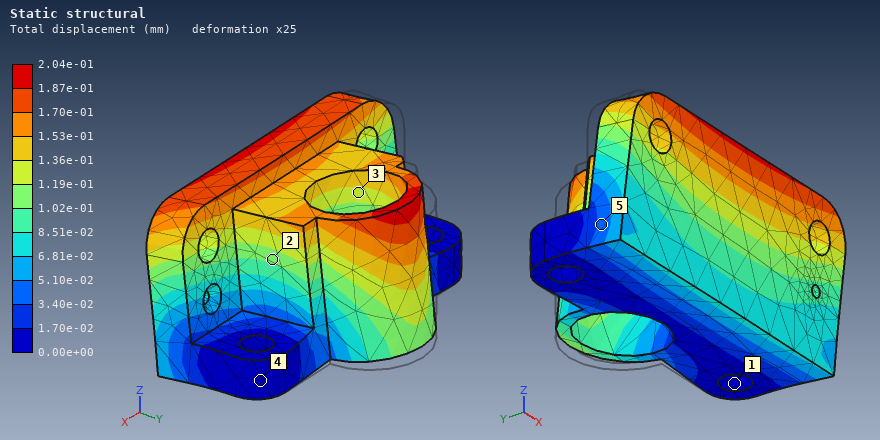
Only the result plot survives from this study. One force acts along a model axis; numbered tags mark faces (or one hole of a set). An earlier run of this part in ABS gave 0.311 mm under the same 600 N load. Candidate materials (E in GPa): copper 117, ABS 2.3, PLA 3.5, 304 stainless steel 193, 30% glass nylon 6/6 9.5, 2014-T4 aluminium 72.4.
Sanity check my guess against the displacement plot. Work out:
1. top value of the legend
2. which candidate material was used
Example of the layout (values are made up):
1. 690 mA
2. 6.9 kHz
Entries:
1. 2.04e-01 mm
2. PLA
